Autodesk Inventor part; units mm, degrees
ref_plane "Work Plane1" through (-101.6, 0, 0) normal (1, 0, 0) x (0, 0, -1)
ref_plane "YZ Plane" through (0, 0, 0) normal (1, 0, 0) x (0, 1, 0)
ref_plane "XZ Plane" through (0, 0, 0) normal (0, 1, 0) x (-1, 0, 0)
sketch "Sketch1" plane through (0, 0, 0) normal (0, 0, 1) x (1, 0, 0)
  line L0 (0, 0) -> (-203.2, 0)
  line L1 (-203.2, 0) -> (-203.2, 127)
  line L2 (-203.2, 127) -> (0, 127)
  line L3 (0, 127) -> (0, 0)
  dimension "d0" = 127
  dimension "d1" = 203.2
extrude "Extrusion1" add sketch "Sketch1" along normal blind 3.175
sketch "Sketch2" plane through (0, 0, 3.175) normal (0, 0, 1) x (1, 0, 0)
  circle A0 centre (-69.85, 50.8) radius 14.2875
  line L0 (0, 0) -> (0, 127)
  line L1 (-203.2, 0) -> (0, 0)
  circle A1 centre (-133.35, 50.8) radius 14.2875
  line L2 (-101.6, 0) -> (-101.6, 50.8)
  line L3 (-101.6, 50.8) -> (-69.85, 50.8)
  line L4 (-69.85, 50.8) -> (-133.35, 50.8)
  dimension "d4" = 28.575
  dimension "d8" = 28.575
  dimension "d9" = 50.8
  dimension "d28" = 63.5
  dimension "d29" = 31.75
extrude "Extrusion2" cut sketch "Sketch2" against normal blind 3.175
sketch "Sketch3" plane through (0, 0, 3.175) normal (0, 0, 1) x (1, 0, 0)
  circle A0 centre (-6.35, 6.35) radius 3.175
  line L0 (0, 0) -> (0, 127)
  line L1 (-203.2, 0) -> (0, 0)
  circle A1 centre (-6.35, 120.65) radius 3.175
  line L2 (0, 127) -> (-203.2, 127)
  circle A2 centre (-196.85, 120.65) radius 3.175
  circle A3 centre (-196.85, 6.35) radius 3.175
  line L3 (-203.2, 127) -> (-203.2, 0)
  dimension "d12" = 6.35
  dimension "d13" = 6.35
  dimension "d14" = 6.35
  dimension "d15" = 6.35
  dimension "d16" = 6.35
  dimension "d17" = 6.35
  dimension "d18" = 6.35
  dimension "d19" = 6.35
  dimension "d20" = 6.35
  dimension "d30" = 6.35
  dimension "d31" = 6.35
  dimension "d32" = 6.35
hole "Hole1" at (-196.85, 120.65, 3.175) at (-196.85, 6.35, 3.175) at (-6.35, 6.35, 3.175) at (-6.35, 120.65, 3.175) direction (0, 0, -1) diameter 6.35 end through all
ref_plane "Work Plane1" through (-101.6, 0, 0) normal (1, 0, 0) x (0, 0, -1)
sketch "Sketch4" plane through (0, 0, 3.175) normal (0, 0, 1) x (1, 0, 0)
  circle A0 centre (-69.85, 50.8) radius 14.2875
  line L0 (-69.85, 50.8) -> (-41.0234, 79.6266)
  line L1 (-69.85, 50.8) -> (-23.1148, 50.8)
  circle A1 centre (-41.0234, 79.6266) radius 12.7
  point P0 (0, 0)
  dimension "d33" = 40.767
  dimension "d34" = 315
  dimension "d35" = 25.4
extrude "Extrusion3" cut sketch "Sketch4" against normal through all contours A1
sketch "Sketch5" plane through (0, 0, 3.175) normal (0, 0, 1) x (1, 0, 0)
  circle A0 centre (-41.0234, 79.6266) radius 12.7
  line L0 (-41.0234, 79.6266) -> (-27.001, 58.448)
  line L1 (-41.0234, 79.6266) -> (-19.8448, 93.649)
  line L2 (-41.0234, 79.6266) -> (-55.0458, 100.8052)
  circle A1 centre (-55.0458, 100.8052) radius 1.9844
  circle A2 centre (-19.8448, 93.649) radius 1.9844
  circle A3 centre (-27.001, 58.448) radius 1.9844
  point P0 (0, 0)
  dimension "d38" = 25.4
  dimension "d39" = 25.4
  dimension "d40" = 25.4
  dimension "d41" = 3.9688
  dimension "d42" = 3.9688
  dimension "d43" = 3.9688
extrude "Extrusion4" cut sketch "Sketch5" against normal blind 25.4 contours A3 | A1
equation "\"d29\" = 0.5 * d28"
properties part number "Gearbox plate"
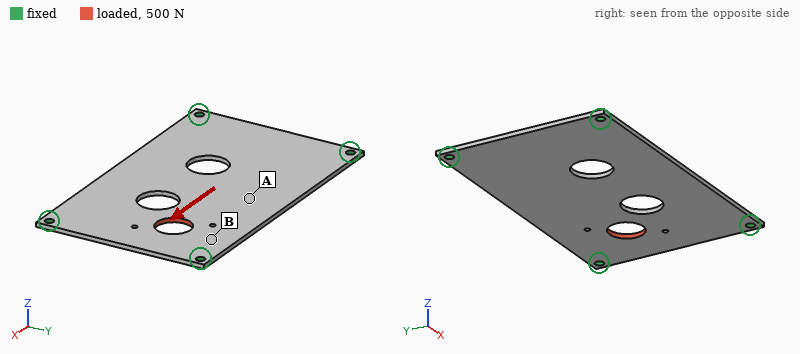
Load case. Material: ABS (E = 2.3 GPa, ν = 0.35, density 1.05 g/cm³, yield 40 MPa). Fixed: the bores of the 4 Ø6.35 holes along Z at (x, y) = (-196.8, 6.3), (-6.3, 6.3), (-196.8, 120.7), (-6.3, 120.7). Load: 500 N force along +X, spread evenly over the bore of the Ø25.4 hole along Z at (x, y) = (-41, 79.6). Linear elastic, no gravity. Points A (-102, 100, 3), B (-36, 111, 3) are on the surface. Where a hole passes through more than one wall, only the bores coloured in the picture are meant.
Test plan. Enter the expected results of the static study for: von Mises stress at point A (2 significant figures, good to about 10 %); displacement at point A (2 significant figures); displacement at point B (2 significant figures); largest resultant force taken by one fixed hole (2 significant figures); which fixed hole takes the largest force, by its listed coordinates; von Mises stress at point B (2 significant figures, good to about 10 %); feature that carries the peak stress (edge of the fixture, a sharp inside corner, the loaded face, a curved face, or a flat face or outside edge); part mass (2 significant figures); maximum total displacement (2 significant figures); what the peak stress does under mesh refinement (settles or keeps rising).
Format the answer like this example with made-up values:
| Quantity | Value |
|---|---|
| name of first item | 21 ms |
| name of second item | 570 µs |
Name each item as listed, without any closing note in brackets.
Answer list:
| Quantity | Value |
|---|---|
| von Mises stress at point A | 0.86 MPa |
| displacement at point A | 0.043 mm |
| displacement at point B | 0.048 mm |
| largest resultant force taken by one fixed hole | 220 N |
| which fixed hole takes the largest force, by its listed coordinates | (-6.3, 120.7) |
| von Mises stress at point B | 1.7 MPa |
| feature that carries the peak stress | edge of the fixture |
| part mass | 80 g |
| maximum total displacement | 0.11 mm |
| what the peak stress does under mesh refinement | keeps rising |
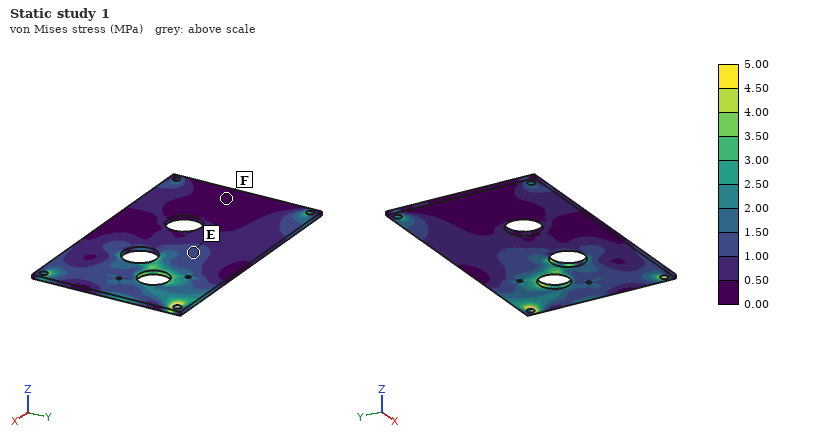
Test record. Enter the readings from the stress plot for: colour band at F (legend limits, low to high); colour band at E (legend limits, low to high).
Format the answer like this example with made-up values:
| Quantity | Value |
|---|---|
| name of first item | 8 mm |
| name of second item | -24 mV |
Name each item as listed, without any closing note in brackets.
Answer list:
| Quantity | Value |
|---|---|
| colour band at F | 0.00 to 0.50 MPa |
| colour band at E | 1.00 to 1.50 MPa |
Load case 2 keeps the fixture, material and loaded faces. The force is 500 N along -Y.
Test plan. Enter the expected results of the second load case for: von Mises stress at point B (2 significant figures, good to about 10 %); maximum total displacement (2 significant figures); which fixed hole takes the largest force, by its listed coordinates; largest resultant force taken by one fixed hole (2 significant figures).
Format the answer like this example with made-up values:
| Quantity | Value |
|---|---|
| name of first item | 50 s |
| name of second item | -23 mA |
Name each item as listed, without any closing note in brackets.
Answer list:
| Quantity | Value |
|---|---|
| von Mises stress at point B | 1.6 MPa |
| maximum total displacement | 0.11 mm |
| which fixed hole takes the largest force, by its listed coordinates | (-6.3, 120.7) |
| largest resultant force taken by one fixed hole | 240 N |
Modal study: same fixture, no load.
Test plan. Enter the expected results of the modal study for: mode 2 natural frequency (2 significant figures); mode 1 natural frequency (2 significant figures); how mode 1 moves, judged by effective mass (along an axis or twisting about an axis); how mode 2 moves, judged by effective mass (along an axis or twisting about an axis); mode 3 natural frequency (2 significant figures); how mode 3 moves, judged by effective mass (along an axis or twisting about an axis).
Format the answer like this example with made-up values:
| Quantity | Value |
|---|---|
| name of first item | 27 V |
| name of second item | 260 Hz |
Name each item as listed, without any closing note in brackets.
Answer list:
| Quantity | Value |
|---|---|
| mode 2 natural frequency | 180 Hz |
| mode 1 natural frequency | 110 Hz |
| how mode 1 moves, judged by effective mass | along Z |
| how mode 2 moves, judged by effective mass | twisting about X |
| mode 3 natural frequency | 280 Hz |
| how mode 3 moves, judged by effective mass | twisting about Y |
